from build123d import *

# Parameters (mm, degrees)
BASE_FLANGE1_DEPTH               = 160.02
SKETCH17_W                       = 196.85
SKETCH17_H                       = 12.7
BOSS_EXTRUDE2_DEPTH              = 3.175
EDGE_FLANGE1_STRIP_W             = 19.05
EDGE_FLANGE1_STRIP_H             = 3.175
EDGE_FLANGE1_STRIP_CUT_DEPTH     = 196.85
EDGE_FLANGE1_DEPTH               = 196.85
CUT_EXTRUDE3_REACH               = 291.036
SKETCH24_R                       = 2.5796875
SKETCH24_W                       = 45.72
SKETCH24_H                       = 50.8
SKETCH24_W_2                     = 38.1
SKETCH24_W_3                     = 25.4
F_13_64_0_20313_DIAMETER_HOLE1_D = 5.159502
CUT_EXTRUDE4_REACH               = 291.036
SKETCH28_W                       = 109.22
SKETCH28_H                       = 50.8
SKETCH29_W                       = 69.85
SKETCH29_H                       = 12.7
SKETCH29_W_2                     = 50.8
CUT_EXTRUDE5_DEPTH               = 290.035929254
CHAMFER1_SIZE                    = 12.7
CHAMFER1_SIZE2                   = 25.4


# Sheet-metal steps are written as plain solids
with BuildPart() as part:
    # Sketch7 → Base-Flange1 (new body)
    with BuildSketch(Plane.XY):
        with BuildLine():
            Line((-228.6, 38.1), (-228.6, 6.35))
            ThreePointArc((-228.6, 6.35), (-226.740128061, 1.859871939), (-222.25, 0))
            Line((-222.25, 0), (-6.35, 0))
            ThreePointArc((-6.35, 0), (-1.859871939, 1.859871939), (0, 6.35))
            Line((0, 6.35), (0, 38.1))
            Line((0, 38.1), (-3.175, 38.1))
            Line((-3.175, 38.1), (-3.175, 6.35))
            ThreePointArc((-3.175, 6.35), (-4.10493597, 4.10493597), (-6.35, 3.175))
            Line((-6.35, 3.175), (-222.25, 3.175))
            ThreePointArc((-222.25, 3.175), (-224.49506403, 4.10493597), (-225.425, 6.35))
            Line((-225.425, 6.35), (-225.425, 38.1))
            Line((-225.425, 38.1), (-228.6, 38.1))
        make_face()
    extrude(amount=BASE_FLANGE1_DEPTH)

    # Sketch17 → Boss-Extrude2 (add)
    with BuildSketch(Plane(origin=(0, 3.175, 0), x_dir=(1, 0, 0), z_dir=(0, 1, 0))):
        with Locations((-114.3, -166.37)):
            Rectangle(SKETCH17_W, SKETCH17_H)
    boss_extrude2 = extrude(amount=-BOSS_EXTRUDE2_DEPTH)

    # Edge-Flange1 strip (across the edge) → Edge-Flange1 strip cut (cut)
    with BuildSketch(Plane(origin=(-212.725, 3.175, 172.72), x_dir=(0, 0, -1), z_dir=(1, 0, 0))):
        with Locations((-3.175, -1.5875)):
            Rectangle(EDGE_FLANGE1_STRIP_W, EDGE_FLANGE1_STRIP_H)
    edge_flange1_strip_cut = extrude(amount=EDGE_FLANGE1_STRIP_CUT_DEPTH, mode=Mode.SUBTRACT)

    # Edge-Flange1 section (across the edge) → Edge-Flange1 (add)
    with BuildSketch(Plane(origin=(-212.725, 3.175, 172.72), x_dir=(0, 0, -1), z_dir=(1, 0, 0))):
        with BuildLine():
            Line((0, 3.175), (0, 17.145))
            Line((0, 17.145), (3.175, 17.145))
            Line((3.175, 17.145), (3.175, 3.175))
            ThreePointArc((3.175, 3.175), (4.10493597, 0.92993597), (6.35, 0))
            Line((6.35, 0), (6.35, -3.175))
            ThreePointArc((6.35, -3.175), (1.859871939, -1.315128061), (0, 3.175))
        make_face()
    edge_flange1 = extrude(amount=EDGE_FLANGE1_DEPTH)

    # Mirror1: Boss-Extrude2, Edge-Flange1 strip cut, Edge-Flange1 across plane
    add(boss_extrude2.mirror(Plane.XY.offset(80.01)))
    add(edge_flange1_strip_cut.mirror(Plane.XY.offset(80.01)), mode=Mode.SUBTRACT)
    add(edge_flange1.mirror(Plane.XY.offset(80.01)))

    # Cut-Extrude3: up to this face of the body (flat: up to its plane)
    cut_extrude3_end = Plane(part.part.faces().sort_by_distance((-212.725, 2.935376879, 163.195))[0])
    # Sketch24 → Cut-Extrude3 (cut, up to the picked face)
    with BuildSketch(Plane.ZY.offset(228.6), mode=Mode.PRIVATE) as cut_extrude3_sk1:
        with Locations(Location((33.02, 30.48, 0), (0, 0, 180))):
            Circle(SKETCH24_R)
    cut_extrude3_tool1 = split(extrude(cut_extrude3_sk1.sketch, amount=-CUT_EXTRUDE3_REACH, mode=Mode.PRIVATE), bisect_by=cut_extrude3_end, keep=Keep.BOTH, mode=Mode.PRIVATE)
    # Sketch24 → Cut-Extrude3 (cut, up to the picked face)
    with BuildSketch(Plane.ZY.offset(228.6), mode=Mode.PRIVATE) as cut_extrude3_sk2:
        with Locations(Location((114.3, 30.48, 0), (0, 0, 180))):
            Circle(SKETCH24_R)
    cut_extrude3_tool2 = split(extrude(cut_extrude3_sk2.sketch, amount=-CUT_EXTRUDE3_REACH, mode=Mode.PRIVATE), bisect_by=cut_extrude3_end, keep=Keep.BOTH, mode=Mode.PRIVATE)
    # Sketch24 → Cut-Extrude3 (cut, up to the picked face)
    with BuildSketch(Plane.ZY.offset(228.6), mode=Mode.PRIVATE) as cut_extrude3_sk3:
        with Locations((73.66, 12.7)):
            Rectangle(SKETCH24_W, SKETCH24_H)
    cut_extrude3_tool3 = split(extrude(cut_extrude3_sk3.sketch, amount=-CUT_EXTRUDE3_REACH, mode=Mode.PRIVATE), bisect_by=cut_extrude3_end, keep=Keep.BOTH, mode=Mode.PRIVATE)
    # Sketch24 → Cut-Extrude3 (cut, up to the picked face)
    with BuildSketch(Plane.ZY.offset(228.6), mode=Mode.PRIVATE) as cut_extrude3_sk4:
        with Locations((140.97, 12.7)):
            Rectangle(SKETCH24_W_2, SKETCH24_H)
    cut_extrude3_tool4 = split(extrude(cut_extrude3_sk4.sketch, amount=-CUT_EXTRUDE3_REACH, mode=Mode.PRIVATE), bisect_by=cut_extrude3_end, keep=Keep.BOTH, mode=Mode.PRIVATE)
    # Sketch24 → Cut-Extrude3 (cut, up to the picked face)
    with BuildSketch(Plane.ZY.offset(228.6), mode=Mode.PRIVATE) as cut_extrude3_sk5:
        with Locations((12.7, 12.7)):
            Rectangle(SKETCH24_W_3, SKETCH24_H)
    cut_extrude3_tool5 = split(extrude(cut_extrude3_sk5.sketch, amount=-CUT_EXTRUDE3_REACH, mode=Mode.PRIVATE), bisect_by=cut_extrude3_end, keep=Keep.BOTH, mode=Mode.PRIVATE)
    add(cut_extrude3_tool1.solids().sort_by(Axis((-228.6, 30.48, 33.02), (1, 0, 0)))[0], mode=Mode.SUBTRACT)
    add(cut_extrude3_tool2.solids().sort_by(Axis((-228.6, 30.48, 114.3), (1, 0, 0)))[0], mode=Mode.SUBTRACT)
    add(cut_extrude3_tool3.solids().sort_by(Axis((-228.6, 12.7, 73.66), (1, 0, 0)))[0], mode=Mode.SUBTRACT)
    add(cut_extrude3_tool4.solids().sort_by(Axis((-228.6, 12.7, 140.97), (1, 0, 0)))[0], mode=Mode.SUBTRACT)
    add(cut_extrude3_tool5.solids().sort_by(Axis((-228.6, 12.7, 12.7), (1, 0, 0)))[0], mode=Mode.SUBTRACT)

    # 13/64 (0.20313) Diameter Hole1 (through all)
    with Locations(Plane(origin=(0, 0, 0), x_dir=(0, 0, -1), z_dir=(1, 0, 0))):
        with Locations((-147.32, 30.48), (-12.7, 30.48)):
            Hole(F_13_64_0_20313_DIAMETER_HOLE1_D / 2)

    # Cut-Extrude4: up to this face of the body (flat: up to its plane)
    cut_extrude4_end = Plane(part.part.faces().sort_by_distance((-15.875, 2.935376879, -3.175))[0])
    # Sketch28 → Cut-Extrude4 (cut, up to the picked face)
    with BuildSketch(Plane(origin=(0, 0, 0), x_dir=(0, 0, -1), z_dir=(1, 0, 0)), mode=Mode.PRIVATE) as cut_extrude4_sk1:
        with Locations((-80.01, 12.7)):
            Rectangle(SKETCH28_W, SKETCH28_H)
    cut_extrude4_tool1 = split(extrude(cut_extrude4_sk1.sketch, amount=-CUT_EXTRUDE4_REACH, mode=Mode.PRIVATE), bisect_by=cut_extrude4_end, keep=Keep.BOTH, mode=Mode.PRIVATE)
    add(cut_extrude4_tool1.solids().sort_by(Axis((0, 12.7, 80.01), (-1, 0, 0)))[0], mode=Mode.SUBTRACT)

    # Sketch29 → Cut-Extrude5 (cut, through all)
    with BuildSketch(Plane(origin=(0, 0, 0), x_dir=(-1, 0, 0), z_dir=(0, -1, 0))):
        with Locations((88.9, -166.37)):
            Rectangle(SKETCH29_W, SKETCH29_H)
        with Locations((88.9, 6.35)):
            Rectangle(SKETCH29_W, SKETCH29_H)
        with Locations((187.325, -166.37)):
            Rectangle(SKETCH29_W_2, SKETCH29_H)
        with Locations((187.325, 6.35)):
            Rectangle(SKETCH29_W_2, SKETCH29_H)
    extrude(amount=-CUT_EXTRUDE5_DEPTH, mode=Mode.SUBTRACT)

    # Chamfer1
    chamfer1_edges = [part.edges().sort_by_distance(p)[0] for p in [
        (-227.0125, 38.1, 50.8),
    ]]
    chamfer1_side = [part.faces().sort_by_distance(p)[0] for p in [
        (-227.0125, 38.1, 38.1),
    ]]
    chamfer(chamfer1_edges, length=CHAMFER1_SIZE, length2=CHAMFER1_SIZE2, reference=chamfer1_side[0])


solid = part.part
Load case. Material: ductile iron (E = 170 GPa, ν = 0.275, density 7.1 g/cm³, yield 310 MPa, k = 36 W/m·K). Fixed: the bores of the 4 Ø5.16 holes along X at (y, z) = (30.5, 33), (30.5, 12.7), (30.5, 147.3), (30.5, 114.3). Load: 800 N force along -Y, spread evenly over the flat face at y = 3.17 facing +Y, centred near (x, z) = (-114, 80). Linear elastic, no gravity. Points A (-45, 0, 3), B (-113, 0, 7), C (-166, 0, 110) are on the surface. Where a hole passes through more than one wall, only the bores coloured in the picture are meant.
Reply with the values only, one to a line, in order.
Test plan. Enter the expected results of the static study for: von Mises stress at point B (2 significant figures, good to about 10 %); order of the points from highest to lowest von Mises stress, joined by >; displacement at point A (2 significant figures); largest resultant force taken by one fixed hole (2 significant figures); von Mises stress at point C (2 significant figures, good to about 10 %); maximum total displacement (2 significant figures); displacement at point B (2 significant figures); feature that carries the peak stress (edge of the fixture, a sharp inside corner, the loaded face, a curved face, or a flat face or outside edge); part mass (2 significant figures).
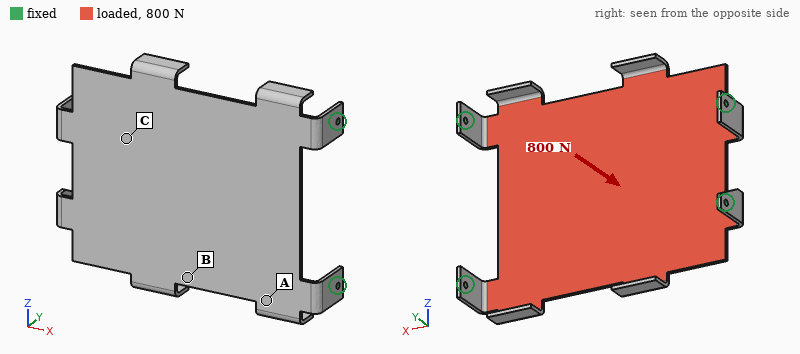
56 MPa
B > C > A
0.33 mm
380 N
31 MPa
0.82 mm
0.71 mm
a curved face
910 g
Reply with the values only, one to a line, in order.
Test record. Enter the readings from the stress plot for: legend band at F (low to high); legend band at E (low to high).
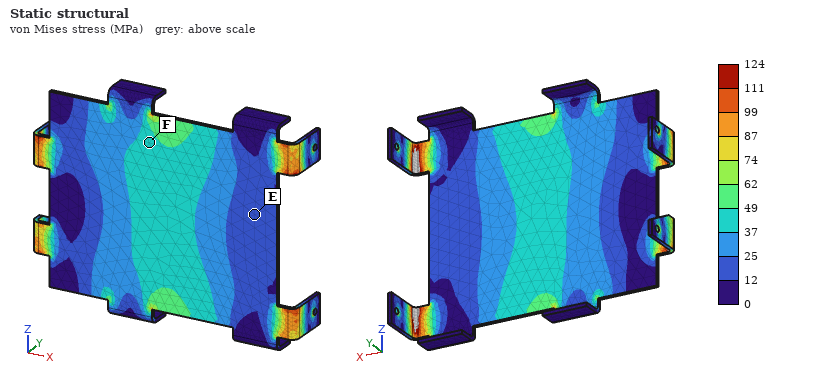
37 to 49 MPa
12 to 25 MPa
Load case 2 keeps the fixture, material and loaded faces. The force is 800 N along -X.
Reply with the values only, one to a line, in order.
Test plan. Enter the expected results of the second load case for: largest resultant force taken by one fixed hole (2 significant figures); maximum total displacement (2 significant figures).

210 N
0.11 mm
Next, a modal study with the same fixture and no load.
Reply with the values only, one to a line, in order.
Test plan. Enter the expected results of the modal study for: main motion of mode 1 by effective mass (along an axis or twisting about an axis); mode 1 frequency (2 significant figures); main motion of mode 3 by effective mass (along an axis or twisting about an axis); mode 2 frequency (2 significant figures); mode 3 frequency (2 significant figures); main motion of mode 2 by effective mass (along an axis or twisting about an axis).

along Y
210 Hz
along X
280 Hz
440 Hz
twisting about X
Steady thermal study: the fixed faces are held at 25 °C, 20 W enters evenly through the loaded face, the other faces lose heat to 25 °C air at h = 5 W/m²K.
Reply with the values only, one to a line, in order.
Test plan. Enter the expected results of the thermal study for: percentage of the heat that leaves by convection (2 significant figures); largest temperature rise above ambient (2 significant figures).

54 %
55 K
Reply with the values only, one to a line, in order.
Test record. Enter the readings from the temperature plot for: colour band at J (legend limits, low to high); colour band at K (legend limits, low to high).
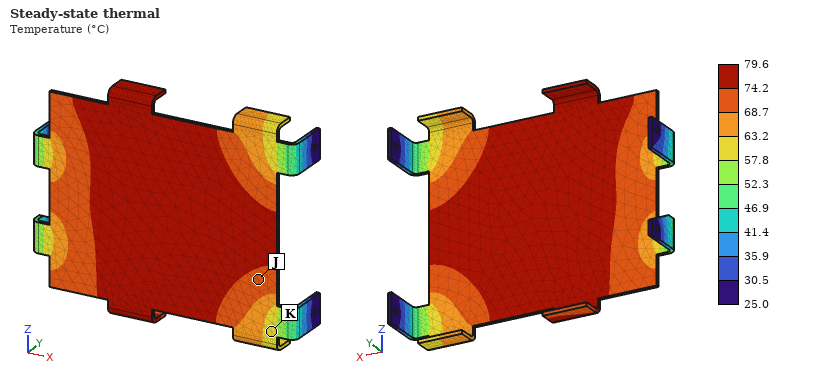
68.7 to 74.2 °C
57.8 to 63.2 °C
